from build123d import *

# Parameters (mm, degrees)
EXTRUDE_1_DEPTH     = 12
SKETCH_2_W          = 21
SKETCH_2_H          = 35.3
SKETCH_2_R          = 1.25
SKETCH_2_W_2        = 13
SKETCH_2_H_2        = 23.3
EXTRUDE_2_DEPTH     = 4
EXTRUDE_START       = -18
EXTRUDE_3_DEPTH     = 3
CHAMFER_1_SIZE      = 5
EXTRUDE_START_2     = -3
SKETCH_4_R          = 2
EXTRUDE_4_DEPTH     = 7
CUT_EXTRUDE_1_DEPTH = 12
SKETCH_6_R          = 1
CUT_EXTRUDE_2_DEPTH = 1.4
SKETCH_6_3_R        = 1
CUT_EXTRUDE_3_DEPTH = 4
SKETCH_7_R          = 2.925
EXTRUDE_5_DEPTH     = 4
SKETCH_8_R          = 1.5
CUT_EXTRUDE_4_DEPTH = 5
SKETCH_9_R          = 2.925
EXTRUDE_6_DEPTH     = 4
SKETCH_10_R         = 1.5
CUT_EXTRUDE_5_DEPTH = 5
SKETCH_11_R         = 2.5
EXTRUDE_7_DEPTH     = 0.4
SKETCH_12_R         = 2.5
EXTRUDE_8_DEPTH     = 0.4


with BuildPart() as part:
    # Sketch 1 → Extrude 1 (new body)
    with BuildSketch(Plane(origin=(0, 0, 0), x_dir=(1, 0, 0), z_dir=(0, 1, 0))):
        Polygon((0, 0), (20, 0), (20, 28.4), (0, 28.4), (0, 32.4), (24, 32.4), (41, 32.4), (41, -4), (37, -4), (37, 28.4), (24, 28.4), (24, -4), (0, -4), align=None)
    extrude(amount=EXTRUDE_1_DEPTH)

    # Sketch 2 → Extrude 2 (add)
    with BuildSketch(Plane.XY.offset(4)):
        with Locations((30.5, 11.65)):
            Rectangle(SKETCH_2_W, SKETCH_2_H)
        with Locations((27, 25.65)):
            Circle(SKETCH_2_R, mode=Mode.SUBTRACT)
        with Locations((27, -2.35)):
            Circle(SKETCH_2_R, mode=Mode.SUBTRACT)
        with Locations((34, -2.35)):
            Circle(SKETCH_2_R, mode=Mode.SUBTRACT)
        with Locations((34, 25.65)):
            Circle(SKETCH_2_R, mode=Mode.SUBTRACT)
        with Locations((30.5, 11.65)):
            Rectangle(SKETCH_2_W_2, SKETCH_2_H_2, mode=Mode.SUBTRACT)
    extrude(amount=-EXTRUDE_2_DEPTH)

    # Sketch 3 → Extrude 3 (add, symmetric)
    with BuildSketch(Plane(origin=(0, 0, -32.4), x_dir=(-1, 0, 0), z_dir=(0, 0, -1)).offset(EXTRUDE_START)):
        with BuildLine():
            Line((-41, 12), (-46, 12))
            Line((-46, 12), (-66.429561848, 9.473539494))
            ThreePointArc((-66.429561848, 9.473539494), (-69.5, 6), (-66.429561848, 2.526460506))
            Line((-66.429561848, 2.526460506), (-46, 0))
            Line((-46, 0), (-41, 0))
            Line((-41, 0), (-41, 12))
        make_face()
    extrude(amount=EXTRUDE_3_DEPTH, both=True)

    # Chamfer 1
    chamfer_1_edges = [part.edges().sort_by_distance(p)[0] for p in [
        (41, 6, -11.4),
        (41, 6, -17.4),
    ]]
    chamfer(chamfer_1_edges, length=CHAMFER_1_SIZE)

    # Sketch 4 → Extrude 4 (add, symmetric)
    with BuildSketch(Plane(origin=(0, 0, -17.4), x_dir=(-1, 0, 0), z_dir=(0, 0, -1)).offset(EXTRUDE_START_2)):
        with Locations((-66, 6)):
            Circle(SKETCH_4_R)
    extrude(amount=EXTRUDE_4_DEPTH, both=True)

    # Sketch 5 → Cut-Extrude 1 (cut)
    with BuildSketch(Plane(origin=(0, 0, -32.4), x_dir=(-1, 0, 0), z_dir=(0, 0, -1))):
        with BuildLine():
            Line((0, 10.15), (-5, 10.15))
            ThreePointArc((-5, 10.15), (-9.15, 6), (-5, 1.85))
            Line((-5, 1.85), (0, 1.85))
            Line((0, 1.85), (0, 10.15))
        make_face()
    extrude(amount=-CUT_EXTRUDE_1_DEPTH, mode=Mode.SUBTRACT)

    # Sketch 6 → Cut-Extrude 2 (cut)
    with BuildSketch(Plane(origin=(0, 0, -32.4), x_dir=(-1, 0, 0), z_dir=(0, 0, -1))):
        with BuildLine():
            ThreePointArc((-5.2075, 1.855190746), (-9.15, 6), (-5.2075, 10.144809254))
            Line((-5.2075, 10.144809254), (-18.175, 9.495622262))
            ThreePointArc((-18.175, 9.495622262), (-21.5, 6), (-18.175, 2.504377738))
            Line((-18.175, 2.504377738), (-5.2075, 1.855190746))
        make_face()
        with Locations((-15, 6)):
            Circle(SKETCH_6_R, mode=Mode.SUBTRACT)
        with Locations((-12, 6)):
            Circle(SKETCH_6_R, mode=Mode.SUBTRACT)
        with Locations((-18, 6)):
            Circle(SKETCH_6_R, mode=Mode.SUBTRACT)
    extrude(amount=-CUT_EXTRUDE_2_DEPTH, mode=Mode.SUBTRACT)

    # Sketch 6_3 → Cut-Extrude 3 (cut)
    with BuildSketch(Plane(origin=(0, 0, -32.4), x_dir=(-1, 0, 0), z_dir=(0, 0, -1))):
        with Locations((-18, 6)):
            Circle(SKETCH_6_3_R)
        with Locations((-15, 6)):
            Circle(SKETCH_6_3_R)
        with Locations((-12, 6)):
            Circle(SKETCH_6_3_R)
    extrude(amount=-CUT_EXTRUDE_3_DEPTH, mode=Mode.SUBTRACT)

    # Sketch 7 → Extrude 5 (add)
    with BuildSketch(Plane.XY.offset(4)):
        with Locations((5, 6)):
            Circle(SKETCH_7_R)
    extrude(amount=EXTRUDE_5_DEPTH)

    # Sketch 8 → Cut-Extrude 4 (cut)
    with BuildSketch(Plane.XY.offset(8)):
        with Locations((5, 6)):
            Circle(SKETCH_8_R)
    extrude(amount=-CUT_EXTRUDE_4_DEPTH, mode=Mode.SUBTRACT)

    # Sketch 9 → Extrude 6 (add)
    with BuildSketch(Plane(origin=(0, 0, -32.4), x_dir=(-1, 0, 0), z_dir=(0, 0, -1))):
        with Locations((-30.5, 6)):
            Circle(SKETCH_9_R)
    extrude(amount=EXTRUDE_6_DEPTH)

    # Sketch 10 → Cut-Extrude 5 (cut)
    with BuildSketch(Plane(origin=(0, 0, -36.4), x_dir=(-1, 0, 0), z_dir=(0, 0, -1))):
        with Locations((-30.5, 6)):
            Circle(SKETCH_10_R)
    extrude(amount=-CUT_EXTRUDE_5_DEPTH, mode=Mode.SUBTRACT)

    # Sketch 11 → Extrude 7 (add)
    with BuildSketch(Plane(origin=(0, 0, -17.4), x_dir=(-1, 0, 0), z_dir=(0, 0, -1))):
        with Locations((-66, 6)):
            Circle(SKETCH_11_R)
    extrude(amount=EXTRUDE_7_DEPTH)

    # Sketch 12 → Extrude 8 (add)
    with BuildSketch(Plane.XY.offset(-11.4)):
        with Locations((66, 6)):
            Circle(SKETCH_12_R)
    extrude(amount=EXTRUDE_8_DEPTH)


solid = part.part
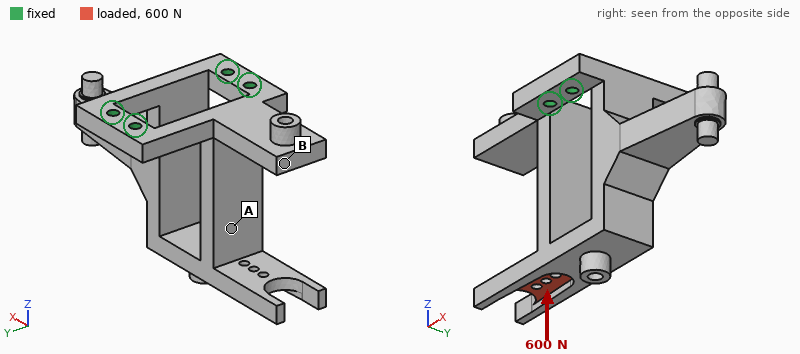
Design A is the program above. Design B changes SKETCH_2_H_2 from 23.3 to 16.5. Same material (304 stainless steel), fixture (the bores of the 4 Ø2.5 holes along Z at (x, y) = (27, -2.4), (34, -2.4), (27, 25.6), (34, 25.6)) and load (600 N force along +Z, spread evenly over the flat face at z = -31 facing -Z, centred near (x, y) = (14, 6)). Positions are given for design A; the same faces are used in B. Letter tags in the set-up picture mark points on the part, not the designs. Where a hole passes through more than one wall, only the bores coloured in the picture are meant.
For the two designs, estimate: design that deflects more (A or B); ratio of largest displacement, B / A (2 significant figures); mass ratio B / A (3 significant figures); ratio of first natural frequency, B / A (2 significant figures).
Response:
A
0.89
1.04
1.1
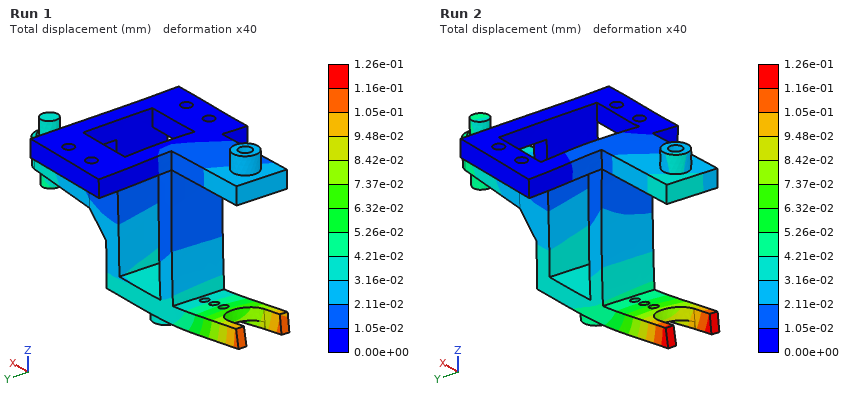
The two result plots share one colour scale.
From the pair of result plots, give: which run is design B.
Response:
Run 1
